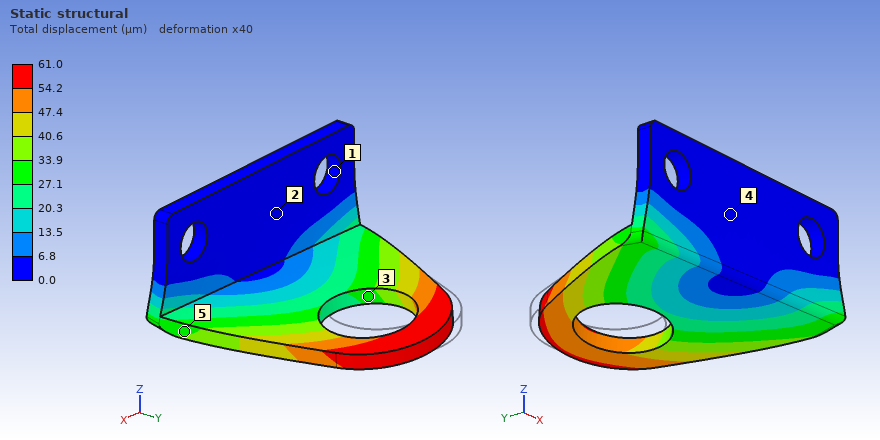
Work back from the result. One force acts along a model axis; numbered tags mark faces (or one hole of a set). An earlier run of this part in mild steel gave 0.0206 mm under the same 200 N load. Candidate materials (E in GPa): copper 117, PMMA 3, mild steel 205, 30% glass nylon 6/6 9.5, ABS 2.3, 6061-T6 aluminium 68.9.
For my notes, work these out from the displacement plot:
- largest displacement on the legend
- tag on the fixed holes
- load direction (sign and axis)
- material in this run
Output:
61.0 µm
1
+X
6061-T6 aluminium
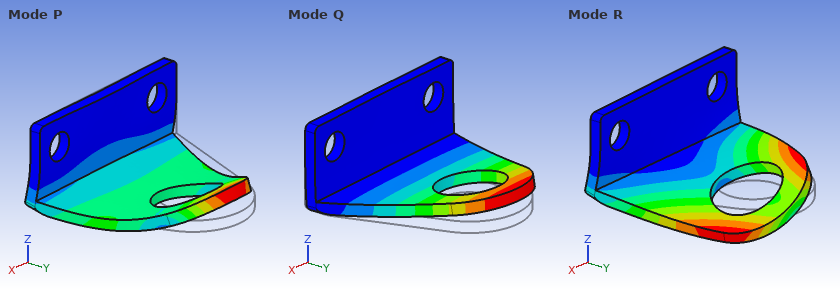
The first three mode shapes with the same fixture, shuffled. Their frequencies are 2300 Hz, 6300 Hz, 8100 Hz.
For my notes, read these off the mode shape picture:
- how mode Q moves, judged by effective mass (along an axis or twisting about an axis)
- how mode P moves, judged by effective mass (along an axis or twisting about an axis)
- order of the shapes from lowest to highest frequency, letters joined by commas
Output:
along Z
along Y
Q, R, P
